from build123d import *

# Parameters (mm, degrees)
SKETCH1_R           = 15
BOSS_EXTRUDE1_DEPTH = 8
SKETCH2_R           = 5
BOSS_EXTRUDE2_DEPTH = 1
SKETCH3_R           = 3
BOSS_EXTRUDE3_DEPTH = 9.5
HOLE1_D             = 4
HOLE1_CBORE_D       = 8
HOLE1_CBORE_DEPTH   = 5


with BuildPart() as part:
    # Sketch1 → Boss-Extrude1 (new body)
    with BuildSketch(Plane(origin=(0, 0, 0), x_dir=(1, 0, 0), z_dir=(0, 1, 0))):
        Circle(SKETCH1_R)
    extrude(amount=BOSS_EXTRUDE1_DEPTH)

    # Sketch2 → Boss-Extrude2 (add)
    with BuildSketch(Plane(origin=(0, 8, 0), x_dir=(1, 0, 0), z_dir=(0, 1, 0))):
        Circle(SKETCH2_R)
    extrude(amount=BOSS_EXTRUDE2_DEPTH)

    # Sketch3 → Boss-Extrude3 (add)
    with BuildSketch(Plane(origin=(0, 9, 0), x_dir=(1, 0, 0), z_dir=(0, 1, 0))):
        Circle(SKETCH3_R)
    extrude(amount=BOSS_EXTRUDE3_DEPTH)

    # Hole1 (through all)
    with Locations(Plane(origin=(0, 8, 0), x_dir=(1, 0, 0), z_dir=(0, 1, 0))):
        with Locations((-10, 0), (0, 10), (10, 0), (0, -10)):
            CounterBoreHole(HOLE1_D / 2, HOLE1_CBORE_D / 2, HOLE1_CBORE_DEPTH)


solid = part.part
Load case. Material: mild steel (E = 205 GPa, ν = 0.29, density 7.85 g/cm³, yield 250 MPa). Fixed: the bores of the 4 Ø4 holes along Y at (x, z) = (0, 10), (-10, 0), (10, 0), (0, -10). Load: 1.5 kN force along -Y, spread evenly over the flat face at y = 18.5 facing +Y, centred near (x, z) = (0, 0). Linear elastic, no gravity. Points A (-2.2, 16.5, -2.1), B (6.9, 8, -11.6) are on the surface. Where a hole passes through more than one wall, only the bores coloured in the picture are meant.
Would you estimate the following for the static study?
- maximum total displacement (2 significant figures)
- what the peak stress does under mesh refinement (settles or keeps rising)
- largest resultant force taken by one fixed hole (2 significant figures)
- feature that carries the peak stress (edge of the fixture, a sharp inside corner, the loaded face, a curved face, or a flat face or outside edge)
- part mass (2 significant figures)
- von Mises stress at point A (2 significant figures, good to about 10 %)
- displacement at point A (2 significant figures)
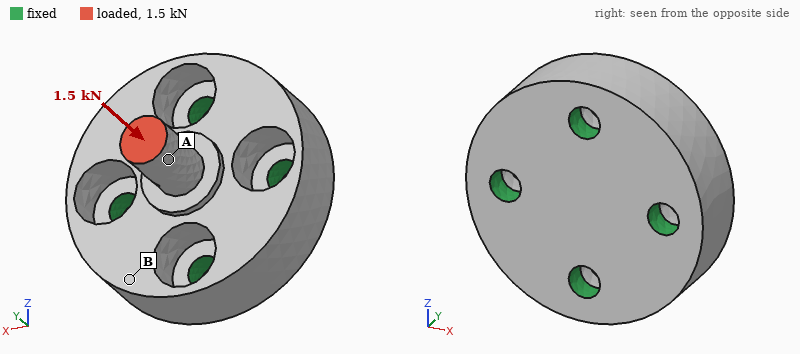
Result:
3.9 µm
keeps rising
410 N
edge of the fixture
38 g
53 MPa
3.4 µm
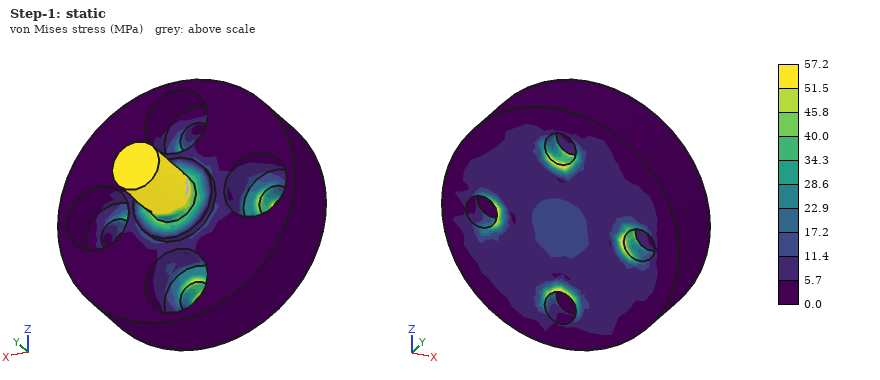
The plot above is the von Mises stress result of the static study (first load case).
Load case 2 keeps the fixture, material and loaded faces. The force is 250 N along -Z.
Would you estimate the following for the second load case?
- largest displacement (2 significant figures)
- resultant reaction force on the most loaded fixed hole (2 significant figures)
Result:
11 µm
220 N
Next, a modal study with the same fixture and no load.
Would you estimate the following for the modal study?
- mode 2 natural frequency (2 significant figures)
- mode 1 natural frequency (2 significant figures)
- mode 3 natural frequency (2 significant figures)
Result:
29 kHz
29 kHz
44 kHz
